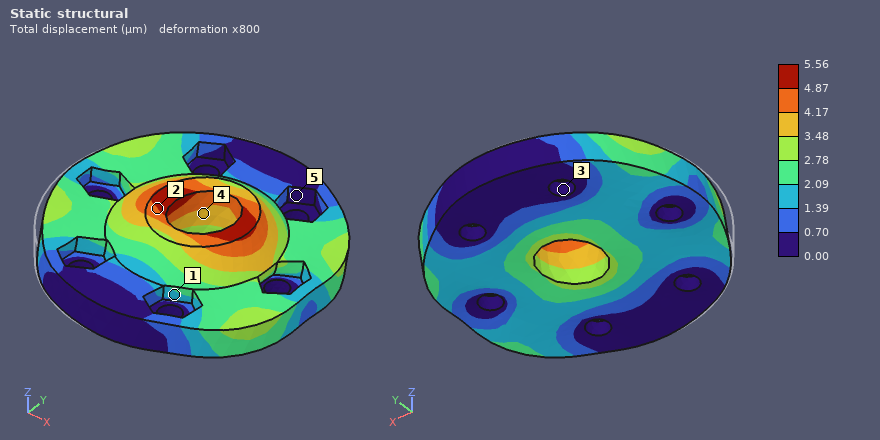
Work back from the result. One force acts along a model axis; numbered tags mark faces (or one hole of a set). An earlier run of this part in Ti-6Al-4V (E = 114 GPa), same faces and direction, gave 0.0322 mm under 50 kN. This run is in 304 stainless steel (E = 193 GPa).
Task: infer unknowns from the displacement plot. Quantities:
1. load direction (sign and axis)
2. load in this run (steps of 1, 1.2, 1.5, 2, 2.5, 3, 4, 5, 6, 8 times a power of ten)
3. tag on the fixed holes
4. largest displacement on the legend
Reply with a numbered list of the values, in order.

1. +X
2. 15 kN
3. 3
4. 5.56 µm
